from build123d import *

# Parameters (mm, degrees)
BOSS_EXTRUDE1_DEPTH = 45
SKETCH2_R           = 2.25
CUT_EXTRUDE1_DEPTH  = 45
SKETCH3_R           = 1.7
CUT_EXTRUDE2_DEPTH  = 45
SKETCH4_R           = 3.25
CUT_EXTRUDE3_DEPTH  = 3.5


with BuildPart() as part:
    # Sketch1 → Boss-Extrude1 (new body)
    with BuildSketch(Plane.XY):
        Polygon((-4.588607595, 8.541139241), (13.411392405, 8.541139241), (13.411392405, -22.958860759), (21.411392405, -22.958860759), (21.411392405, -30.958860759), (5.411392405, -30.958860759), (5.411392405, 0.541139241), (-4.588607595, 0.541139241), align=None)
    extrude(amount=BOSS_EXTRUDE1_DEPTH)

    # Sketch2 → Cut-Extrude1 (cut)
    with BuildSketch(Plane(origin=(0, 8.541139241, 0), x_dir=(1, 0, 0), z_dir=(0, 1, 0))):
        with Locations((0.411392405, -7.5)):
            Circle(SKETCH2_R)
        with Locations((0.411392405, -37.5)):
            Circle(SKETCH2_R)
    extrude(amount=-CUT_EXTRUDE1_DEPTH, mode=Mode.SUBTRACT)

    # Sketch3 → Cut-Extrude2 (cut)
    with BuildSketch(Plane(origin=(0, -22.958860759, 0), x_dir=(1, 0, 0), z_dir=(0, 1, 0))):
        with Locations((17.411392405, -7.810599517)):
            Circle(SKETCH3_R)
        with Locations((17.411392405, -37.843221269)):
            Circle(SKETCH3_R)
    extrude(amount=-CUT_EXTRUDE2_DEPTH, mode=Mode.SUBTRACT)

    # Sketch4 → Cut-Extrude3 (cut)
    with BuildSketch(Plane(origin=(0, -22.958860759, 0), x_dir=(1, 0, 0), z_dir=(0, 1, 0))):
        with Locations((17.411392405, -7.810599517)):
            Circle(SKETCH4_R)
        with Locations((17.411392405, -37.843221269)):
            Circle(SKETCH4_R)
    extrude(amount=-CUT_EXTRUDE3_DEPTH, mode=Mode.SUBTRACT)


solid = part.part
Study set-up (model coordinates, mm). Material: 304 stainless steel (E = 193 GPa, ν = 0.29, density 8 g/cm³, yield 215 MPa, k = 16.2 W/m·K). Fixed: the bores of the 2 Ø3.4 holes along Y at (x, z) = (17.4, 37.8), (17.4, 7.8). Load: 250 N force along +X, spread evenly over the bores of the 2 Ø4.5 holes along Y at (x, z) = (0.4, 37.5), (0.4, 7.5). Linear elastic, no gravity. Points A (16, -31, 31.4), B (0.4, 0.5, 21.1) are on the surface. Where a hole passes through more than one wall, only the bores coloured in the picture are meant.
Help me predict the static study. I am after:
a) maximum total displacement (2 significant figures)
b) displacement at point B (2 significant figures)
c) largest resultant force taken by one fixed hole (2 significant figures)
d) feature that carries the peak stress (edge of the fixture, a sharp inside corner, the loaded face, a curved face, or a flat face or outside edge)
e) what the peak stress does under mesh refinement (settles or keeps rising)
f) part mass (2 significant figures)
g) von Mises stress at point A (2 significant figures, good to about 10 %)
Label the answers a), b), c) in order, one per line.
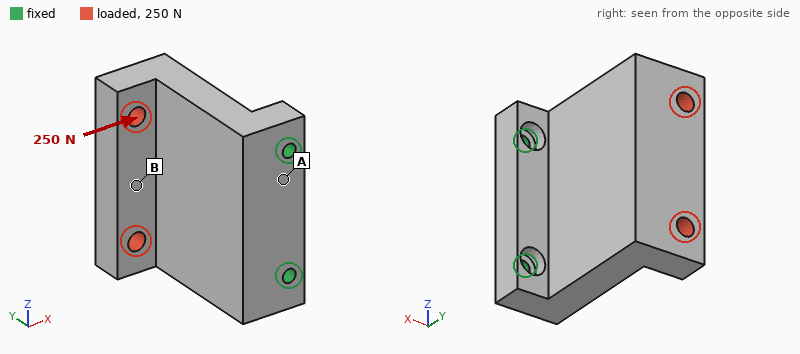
a) 32 µm
b) 24 µm
c) 150 N
d) edge of the fixture
e) keeps rising
f) 160 g
g) 16 MPa
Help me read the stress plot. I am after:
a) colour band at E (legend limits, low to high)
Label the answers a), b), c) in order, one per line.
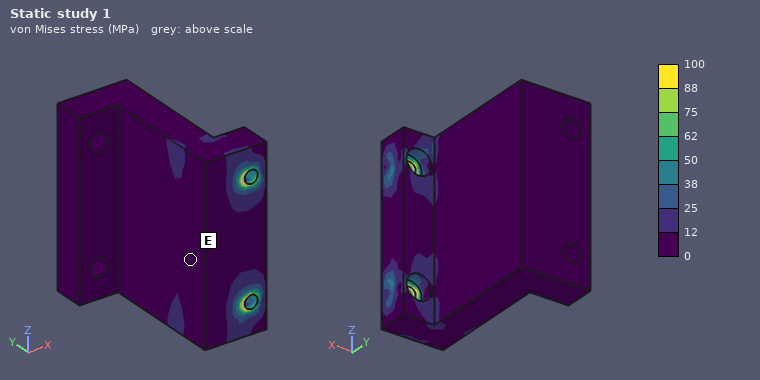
a) 0 to 12 MPa
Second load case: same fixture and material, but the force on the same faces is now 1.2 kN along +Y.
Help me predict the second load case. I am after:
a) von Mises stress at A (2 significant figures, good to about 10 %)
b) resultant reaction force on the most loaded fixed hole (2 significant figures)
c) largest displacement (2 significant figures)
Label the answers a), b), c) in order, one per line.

a) 33 MPa
b) 620 N
c) 76 µm
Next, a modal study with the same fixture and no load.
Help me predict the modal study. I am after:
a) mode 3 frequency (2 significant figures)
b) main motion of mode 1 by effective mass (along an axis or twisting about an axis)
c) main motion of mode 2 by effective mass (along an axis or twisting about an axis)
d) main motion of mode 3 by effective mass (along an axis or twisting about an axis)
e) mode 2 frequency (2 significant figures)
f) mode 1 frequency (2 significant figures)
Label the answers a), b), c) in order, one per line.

a) 6900 Hz
b) along X
c) along Z
d) along Z
e) 5900 Hz
f) 1800 Hz
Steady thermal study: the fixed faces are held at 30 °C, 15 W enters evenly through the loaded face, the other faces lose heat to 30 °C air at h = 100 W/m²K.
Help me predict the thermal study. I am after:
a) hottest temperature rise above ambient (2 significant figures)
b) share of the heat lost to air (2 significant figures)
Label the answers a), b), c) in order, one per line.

a) 55 K
b) 84 %
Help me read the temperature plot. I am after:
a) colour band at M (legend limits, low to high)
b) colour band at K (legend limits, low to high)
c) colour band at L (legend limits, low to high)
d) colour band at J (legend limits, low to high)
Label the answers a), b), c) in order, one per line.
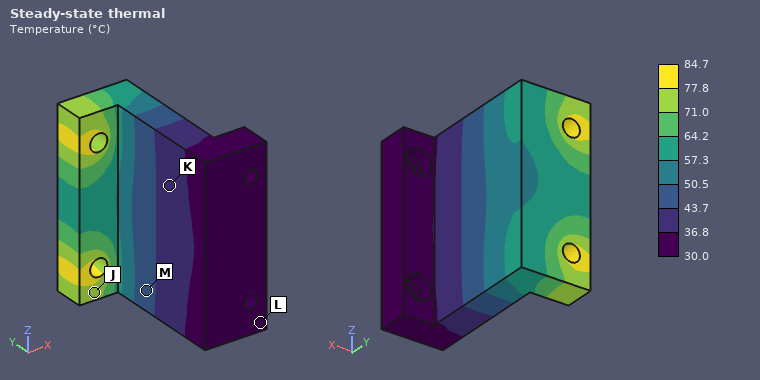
a) 43.7 to 50.5 °C
b) 36.8 to 43.7 °C
c) 30.0 to 36.8 °C
d) 71.0 to 77.8 °C
